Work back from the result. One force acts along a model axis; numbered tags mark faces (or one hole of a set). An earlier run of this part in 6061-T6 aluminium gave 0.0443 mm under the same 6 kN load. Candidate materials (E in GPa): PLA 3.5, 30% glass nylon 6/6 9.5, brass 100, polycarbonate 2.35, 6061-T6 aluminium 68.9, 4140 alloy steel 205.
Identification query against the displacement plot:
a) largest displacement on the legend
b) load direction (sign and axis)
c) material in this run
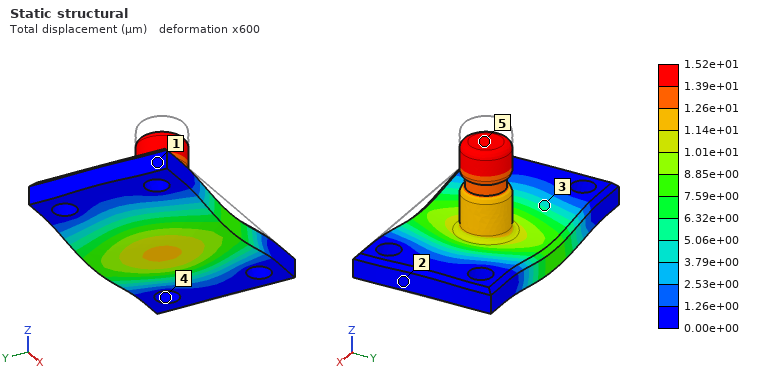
1.52e+01 µm
-Z
4140 alloy steel
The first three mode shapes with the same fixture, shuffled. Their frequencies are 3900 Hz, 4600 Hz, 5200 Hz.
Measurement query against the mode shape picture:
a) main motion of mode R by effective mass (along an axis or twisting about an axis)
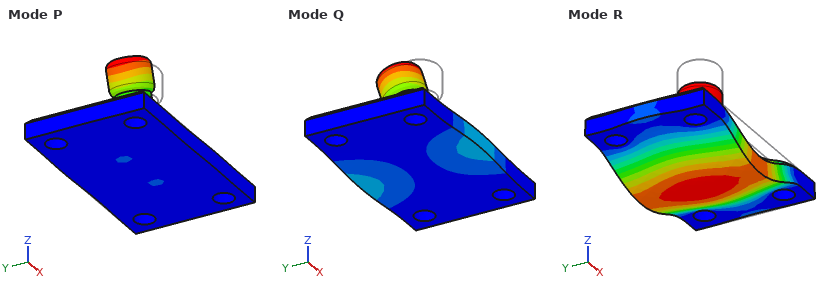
along Z
